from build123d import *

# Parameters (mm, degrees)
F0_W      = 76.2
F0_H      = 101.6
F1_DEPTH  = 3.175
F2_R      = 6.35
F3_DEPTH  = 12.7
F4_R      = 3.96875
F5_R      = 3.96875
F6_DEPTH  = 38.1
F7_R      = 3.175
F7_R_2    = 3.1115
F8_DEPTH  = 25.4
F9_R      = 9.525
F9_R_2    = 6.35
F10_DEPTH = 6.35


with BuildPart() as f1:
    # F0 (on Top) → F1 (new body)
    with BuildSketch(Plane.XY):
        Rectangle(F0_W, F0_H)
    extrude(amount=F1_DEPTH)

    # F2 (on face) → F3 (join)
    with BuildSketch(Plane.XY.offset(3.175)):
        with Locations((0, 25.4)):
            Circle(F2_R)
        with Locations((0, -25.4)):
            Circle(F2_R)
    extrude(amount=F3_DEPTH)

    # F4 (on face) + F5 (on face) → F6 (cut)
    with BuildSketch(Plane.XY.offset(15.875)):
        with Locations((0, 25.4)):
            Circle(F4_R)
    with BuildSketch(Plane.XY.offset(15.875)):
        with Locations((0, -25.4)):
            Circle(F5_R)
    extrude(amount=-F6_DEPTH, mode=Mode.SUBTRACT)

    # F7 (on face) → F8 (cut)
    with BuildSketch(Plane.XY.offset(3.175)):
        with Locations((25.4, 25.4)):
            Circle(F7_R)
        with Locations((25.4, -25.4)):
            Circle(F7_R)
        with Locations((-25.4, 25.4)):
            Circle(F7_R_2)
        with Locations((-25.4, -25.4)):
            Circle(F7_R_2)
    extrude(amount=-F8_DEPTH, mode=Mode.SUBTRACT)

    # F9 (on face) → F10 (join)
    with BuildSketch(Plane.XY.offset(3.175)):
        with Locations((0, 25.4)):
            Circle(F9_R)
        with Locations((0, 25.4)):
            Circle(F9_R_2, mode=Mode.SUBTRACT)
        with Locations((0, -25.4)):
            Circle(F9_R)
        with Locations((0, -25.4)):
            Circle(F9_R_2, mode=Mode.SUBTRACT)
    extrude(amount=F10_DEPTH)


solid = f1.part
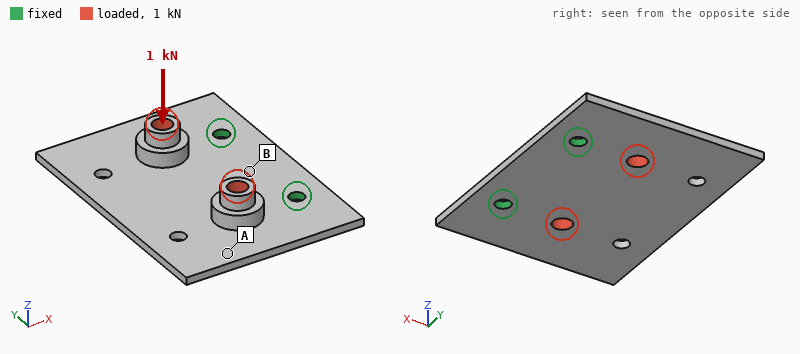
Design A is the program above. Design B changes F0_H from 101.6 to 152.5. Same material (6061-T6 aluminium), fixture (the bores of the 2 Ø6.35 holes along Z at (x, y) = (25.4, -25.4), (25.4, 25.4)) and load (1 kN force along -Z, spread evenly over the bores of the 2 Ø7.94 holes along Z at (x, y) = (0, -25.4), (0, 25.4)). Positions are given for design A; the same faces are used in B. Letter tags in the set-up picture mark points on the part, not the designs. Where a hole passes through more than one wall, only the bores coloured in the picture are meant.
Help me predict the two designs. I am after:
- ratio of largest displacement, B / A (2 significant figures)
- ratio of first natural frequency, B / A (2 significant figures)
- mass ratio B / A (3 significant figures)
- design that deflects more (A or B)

0.92
0.84
1.44
A
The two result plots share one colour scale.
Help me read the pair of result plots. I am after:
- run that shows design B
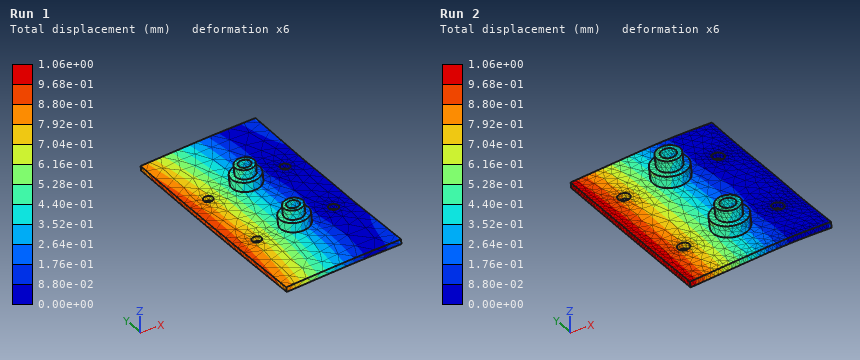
Run 1
